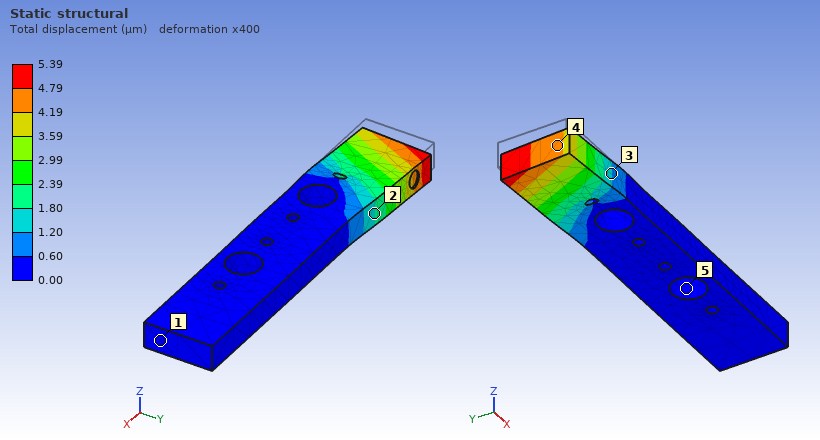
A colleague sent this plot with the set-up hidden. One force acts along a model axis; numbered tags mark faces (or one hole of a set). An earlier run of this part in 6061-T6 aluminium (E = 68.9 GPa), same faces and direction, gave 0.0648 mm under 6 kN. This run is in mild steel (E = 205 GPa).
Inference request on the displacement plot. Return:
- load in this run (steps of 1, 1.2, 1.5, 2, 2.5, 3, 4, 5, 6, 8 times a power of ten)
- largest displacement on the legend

1.5 kN
5.39 µm
